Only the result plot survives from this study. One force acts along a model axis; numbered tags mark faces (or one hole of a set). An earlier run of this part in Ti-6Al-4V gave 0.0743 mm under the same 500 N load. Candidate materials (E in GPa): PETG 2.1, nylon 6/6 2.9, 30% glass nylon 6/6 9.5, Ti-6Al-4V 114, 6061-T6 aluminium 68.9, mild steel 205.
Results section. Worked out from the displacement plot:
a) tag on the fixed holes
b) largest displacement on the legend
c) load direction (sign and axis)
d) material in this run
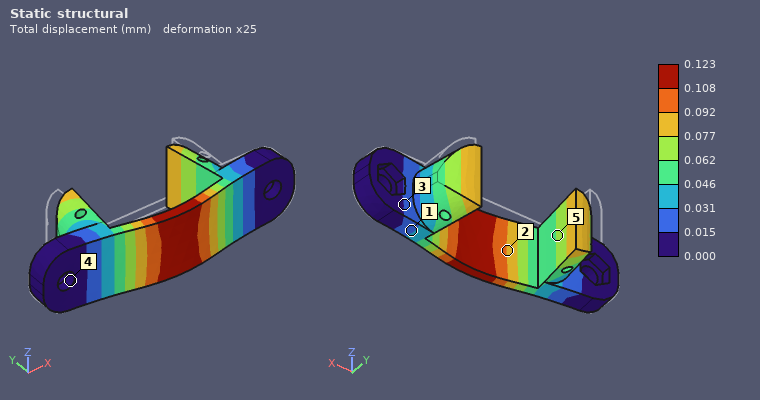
4
0.123 mm
-Y
6061-T6 aluminium
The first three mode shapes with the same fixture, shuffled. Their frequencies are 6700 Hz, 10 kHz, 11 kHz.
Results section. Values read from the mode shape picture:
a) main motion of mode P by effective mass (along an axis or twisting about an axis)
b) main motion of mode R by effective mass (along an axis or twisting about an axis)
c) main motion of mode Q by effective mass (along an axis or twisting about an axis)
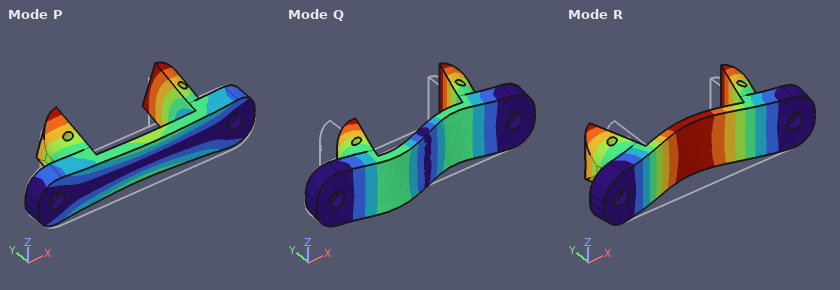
along Z
along Y
along X
